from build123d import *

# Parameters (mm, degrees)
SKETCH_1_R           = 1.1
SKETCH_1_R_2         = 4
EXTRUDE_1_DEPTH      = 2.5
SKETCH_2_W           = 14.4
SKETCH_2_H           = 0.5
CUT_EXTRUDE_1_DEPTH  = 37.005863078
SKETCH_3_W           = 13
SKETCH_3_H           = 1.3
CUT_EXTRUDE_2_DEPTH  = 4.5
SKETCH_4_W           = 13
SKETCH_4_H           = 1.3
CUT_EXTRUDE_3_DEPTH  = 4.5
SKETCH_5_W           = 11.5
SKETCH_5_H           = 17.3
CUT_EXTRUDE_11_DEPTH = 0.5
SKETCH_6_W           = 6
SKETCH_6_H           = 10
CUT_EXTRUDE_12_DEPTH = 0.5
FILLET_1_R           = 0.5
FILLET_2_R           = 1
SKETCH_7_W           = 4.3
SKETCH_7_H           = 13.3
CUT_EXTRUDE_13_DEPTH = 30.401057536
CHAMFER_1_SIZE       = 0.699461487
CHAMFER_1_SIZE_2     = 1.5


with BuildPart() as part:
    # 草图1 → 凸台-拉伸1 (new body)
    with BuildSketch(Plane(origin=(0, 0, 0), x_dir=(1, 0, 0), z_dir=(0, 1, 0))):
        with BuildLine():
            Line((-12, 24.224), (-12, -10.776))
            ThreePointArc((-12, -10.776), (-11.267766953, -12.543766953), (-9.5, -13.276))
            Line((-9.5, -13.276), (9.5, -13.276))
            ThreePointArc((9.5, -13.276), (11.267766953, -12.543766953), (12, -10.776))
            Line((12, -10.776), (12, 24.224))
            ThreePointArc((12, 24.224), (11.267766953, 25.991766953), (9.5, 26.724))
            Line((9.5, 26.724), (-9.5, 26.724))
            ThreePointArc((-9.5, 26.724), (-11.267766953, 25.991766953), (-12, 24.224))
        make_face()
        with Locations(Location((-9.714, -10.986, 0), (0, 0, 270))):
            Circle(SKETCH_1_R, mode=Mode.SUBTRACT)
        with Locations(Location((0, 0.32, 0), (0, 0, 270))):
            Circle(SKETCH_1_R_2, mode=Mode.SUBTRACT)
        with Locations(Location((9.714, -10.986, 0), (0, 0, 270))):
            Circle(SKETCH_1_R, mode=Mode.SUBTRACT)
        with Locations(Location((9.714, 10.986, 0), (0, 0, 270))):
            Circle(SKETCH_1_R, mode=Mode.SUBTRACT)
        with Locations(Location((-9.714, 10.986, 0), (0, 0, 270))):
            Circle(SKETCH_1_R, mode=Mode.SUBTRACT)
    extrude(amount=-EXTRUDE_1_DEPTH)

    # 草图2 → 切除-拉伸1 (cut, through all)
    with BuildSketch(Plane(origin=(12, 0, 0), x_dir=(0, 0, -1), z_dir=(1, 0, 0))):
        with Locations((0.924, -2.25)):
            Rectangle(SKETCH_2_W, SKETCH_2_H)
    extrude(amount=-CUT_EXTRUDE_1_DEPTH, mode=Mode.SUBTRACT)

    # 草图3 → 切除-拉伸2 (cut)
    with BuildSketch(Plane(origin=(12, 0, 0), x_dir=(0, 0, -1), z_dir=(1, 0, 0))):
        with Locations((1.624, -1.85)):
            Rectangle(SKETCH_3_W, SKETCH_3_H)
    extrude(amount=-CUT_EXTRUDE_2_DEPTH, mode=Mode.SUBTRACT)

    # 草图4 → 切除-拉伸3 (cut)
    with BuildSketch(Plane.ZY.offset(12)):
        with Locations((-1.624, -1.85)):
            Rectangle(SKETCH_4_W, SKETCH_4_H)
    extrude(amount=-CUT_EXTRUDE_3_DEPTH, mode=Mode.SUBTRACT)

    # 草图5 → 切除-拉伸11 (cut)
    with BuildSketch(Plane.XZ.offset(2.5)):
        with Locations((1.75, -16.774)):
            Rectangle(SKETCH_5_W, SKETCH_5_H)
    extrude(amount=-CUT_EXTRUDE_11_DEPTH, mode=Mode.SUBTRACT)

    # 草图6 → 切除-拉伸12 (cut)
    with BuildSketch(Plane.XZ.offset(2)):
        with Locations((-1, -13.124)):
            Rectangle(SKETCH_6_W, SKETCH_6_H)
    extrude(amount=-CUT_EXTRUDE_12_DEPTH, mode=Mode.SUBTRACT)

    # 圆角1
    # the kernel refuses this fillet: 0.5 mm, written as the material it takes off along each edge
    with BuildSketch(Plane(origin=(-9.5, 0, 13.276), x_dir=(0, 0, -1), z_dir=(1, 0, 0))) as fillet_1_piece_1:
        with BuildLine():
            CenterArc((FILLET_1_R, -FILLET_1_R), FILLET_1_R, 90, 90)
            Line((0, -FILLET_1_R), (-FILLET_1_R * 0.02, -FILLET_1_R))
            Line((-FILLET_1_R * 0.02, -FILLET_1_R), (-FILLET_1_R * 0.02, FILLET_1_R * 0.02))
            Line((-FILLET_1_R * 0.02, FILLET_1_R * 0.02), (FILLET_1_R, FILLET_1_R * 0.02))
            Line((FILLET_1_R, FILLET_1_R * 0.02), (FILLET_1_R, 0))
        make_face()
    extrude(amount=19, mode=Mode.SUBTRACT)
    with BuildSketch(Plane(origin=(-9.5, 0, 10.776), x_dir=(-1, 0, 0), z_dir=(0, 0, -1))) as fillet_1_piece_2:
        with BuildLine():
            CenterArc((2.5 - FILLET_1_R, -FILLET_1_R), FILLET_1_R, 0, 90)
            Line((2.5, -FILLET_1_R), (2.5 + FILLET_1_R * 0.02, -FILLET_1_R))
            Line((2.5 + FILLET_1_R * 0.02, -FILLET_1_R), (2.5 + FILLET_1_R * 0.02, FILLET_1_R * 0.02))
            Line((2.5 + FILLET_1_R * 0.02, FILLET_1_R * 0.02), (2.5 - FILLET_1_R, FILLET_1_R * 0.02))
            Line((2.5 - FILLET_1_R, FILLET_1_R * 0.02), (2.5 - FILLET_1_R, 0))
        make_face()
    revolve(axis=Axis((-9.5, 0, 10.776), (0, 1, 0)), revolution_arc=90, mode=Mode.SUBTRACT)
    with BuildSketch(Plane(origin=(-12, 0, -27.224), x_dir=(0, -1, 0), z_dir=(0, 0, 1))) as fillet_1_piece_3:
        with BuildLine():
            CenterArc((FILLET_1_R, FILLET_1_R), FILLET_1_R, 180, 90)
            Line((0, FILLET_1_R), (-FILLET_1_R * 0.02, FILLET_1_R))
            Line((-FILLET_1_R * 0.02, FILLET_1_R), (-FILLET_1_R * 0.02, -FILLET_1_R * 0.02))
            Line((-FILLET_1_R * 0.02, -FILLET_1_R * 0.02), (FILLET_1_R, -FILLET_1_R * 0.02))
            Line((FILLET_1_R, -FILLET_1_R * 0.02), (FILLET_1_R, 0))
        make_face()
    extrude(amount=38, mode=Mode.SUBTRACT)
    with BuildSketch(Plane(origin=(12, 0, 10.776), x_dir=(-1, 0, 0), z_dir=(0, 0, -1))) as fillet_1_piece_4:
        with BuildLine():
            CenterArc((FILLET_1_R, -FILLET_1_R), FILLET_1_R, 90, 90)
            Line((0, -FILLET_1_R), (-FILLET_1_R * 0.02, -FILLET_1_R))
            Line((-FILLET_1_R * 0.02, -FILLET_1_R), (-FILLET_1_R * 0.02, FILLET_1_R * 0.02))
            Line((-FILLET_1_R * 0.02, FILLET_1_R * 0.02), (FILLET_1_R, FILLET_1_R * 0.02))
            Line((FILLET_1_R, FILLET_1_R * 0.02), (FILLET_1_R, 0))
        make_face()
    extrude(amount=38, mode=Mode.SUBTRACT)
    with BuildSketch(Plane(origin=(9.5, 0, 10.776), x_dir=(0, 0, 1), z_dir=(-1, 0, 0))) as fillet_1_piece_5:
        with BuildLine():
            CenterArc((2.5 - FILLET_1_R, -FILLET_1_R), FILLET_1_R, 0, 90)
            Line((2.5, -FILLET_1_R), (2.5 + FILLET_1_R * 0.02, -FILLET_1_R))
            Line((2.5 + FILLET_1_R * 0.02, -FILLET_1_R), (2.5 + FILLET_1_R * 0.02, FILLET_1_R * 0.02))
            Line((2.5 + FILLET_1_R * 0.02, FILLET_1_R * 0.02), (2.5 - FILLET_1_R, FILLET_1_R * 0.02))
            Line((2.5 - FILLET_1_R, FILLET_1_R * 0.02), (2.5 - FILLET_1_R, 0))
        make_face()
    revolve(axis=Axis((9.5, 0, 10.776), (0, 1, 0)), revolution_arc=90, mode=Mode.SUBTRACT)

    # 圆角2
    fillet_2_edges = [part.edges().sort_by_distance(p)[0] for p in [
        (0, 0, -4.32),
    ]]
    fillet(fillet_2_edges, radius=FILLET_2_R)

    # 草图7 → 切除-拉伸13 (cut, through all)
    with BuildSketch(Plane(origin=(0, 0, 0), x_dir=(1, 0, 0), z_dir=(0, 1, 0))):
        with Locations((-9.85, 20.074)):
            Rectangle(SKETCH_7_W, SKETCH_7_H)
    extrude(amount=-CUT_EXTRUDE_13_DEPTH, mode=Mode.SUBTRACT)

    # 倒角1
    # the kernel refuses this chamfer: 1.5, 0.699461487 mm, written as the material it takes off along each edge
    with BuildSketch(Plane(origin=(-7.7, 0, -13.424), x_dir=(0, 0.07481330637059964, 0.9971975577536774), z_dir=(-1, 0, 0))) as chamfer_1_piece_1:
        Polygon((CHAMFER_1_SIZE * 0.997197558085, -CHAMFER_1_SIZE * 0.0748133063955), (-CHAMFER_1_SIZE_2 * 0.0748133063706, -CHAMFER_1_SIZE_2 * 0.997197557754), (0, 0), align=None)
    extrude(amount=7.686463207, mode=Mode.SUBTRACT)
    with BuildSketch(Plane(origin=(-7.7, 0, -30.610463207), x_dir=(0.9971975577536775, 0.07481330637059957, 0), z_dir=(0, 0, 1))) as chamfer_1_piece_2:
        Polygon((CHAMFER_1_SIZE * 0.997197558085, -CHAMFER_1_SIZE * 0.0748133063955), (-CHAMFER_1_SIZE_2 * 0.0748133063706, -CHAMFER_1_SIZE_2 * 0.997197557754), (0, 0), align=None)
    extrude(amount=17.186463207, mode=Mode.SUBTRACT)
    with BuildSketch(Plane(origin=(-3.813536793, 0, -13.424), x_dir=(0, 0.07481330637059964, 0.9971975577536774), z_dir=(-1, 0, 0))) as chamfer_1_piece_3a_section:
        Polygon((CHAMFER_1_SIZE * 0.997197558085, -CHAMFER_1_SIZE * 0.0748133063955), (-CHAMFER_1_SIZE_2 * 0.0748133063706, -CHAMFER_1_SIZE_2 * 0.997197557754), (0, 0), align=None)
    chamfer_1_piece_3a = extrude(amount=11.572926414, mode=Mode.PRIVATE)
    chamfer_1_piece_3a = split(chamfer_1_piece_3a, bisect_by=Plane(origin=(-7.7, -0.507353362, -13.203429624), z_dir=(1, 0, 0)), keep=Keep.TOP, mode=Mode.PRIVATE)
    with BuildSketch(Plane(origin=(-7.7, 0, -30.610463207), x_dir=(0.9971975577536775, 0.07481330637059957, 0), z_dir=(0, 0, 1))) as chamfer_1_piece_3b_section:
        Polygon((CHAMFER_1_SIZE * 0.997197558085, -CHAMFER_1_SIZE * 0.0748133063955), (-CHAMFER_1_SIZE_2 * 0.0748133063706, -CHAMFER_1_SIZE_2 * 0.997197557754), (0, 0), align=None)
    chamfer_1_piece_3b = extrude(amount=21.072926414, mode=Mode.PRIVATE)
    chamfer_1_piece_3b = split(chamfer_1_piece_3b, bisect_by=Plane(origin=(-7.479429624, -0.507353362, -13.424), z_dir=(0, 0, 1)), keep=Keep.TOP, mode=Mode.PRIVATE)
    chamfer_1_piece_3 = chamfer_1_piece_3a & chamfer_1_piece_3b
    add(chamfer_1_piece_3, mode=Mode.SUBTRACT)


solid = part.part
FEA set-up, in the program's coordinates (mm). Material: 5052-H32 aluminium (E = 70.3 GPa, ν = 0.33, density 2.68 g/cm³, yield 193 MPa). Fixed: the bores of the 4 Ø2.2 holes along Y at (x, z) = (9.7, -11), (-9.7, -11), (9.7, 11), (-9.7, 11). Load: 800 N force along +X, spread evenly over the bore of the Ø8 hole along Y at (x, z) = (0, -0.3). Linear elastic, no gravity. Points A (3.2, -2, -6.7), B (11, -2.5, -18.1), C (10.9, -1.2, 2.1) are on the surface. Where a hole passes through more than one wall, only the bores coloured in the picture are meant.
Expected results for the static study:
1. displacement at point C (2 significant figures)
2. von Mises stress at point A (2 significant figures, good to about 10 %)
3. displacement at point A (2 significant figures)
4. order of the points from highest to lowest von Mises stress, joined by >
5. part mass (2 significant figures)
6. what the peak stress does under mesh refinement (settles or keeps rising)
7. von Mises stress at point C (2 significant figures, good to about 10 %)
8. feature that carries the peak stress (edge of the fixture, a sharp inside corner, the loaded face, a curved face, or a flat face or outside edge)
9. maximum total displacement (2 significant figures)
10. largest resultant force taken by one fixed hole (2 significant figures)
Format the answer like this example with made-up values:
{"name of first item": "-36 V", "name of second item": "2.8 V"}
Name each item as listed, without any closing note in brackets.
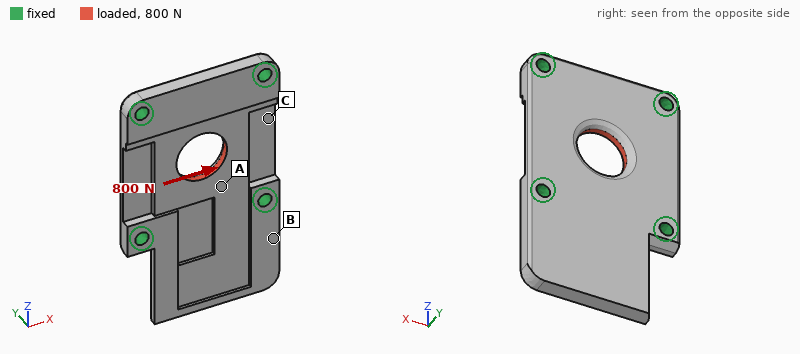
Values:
{"displacement at point C": "3.9 µm", "von Mises stress at point A": "20 MPa", "displacement at point A": "2.4 µm", "order of the points from highest to lowest von Mises stress, joined by >": "A > C > B", "part mass": "4.5 g", "what the peak stress does under mesh refinement": "keeps rising", "von Mises stress at point C": "10 MPa", "feature that carries the peak stress": "edge of the fixture", "maximum total displacement": "5.7 µm", "largest resultant force taken by one fixed hole": "240 N"}
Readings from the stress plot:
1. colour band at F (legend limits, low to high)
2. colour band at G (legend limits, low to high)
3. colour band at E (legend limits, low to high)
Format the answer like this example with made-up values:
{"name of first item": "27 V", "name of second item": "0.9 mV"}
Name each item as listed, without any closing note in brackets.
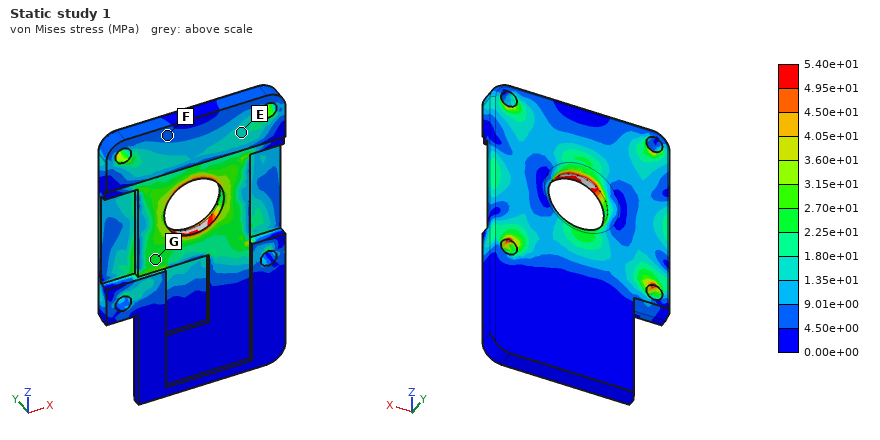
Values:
{"colour band at F": "4.50e+00 to 9.01e+00 MPa", "colour band at G": "2.25e+01 to 2.70e+01 MPa", "colour band at E": "1.35e+01 to 1.80e+01 MPa"}
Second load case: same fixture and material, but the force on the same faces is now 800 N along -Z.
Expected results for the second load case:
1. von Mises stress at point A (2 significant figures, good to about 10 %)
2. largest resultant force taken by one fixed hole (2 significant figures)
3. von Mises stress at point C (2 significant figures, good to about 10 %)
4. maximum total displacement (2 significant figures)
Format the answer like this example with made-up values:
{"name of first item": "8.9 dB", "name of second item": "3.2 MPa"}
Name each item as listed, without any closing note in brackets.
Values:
{"von Mises stress at point A": "23 MPa", "largest resultant force taken by one fixed hole": "220 N", "von Mises stress at point C": "8.6 MPa", "maximum total displacement": "4.9 µm"}
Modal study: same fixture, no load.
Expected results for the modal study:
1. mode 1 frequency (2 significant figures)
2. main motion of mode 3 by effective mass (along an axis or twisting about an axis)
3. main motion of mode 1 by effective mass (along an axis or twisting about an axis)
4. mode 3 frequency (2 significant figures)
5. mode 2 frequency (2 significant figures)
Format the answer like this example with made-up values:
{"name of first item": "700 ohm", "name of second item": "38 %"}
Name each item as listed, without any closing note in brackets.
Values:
{"mode 1 frequency": "6600 Hz", "main motion of mode 3 by effective mass": "along Y", "main motion of mode 1 by effective mass": "along Y", "mode 3 frequency": "20 kHz", "mode 2 frequency": "14 kHz"}
